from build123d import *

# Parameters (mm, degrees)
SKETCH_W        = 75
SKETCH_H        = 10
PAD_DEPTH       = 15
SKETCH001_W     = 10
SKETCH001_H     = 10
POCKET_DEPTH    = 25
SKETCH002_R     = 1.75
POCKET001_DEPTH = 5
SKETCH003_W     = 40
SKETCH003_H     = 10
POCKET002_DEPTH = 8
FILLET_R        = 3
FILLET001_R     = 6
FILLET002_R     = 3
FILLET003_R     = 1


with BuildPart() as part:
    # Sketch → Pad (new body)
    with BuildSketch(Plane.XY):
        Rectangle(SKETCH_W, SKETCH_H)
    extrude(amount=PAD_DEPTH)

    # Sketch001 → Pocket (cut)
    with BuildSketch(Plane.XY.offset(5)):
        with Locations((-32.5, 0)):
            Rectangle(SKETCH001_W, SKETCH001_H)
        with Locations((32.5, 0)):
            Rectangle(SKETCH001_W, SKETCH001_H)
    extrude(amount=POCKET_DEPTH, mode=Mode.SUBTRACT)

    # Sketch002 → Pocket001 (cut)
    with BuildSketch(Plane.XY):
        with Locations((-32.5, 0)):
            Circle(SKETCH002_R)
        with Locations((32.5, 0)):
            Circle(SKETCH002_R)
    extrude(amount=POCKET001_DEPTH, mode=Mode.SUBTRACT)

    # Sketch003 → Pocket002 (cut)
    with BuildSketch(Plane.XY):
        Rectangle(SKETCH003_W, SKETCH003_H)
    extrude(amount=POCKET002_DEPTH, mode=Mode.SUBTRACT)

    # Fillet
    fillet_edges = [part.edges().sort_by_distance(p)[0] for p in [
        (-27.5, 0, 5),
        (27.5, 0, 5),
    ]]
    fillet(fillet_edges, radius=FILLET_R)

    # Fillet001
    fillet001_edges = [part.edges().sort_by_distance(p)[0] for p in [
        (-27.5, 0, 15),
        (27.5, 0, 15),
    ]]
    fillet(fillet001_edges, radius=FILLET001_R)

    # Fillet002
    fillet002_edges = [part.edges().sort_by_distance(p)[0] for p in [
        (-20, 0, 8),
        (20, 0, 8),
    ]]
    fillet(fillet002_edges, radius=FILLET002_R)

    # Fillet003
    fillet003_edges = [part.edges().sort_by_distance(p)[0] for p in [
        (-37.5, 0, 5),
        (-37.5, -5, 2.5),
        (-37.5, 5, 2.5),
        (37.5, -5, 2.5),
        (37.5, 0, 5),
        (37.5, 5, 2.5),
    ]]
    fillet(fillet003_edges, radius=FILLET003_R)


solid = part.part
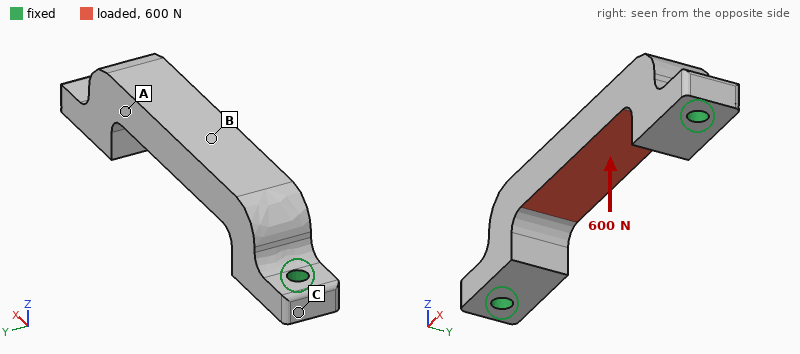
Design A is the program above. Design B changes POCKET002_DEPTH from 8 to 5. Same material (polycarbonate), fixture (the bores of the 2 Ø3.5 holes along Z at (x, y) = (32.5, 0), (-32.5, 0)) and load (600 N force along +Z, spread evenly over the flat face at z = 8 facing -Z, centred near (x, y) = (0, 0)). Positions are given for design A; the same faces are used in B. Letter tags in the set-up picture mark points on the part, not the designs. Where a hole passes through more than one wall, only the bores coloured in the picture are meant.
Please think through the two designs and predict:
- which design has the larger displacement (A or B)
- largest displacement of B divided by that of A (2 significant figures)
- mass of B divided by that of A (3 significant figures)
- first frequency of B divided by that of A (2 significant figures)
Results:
A
0.69
1.20
0.95
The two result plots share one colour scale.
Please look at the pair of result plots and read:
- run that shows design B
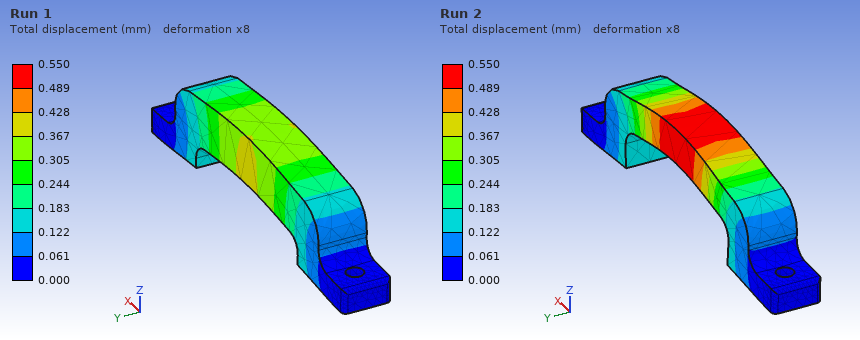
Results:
Run 1
